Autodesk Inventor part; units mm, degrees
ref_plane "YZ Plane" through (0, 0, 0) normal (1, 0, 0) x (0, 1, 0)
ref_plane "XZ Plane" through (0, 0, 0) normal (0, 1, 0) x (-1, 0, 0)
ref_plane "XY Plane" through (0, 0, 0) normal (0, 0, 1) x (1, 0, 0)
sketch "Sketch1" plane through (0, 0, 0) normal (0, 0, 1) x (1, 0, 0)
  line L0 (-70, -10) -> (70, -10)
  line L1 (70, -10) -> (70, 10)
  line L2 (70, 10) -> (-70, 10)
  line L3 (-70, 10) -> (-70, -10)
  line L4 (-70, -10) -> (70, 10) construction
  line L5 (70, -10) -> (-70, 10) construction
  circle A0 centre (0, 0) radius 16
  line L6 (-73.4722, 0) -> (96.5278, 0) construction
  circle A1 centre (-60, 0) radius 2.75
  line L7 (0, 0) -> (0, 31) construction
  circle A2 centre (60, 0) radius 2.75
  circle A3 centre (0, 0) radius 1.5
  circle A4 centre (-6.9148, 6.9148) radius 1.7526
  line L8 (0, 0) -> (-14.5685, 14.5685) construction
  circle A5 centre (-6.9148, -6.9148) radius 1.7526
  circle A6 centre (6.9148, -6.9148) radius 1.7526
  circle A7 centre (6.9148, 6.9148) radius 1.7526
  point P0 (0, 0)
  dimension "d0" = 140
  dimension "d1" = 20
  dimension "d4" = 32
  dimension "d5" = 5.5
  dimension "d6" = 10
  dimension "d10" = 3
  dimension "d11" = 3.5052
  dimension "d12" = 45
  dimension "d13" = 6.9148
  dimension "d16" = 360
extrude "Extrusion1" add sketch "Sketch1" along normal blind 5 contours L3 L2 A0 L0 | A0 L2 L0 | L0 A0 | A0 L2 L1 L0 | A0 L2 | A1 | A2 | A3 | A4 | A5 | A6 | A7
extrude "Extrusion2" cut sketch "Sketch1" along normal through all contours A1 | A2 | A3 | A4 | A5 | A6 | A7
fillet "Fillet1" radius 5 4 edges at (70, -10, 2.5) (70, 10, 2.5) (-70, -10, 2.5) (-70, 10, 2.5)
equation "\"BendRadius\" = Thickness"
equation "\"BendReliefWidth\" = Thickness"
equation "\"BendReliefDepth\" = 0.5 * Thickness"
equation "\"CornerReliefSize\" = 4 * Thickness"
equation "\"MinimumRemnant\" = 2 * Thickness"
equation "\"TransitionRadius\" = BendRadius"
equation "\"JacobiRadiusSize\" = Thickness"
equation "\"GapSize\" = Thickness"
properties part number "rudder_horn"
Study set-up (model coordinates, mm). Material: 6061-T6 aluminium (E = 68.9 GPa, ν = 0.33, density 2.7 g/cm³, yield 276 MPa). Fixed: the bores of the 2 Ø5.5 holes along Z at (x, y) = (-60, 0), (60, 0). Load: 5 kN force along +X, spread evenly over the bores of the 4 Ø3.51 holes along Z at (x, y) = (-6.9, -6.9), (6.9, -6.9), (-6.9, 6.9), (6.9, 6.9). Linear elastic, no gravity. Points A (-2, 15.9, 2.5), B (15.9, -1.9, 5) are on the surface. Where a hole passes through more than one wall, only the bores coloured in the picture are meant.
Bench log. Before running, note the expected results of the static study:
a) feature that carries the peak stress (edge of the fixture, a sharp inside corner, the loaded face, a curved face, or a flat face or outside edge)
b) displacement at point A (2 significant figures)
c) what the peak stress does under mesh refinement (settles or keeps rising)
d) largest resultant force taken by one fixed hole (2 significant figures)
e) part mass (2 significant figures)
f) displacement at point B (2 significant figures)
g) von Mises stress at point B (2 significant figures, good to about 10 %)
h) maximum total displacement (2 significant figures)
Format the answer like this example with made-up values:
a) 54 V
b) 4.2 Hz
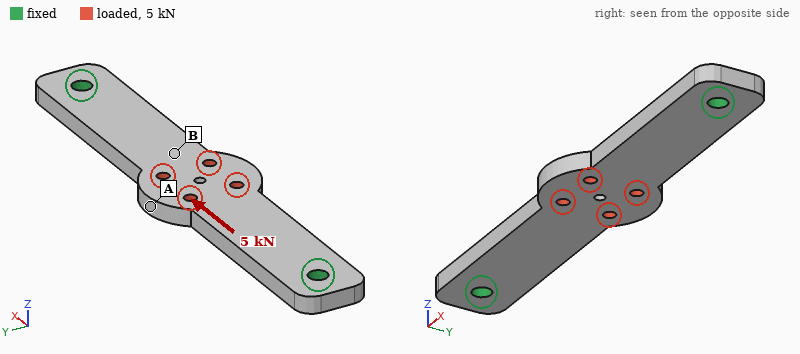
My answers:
a) edge of the fixture
b) 20 µm
c) keeps rising
d) 2.5 kN
e) 39 g
f) 17 µm
g) 22 MPa
h) 22 µm
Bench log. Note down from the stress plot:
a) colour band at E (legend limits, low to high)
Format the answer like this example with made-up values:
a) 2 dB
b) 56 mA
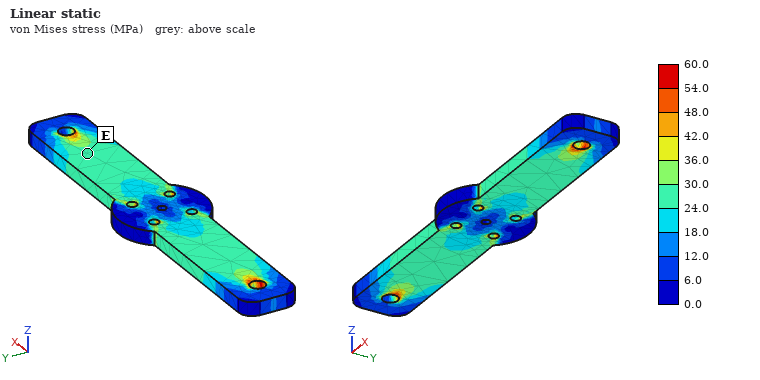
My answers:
a) 24.0 to 30.0 MPa
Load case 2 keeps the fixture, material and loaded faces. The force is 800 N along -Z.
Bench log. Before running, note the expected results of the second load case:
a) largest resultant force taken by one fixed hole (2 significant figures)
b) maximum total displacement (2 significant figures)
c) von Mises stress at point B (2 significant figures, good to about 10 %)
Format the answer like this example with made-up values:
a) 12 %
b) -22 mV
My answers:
a) 400 N
b) 0.46 mm
c) 69 MPa
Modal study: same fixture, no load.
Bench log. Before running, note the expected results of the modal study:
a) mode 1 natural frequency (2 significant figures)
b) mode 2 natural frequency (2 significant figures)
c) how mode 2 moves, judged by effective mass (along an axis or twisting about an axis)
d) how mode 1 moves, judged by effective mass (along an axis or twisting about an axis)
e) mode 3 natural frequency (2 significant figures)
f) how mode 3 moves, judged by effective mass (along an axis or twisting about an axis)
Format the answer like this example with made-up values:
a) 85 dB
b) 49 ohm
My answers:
a) 1700 Hz
b) 4500 Hz
c) twisting about X
d) along Z
e) 4800 Hz
f) along Y
